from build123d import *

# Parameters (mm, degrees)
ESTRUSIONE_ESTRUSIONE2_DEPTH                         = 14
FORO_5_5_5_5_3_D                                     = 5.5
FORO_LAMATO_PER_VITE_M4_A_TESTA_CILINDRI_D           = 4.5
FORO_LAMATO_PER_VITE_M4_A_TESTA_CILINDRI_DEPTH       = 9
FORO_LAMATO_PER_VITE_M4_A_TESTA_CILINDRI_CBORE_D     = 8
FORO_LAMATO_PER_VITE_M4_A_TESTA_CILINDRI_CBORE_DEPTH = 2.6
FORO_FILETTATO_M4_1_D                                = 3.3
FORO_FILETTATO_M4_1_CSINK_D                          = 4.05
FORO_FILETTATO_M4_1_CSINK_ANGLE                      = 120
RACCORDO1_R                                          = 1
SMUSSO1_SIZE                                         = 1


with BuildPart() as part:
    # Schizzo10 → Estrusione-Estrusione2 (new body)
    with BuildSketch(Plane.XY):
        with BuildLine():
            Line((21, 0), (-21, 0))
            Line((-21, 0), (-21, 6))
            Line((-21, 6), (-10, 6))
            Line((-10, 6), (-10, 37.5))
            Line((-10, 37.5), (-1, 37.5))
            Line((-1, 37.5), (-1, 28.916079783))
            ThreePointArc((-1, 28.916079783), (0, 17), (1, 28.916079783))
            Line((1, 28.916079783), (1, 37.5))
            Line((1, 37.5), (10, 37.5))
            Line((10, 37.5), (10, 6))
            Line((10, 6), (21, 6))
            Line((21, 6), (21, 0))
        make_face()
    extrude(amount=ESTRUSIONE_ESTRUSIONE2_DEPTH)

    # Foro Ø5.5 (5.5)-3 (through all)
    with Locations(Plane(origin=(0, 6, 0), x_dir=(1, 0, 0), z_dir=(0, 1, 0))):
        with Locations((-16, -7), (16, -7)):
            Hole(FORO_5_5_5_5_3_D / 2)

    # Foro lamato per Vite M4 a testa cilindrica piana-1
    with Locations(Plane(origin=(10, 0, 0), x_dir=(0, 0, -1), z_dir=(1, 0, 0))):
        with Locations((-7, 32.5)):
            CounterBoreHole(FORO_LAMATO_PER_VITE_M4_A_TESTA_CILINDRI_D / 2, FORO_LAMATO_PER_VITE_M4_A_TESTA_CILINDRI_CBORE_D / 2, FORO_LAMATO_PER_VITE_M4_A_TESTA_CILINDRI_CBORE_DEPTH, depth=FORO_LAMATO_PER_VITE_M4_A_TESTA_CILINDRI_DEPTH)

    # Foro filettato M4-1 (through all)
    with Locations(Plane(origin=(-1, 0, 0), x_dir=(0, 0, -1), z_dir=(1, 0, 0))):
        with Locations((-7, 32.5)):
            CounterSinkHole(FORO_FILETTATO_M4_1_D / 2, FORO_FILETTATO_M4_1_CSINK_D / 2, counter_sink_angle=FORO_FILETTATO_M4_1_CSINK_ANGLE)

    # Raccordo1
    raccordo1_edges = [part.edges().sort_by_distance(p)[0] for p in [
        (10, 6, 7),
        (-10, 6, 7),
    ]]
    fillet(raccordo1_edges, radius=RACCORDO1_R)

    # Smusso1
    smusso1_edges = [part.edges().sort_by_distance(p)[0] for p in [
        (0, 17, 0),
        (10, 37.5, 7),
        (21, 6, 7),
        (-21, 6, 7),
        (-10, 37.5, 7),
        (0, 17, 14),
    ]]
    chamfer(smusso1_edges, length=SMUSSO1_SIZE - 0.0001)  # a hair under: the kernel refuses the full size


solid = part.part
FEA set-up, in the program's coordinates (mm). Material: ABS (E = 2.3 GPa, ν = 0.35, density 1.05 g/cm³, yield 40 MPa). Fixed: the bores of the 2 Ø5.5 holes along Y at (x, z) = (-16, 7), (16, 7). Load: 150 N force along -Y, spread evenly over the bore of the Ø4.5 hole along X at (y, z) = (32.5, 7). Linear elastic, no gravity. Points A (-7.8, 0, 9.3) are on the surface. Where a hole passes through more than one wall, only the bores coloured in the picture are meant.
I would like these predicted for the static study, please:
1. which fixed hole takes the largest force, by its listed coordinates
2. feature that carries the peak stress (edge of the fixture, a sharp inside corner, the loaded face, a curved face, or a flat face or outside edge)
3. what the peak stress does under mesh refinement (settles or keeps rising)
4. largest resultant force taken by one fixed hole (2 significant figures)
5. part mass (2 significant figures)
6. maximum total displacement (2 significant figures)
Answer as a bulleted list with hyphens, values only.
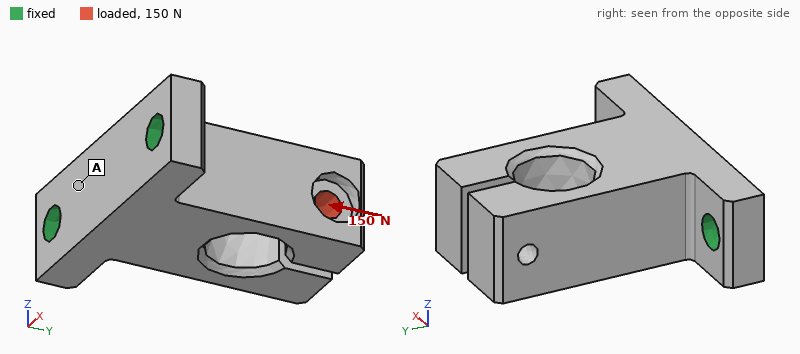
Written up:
- (16, 7)
- a sharp inside corner
- keeps rising
- 110 N
- 10 g
- 0.43 mm
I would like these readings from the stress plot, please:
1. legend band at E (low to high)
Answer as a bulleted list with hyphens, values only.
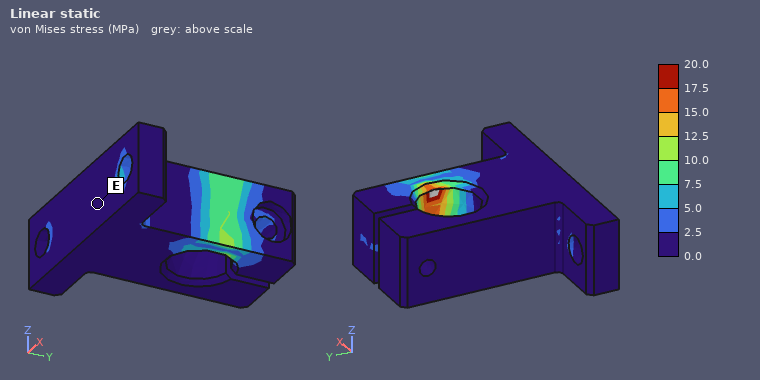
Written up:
- 0.0 to 2.5 MPa
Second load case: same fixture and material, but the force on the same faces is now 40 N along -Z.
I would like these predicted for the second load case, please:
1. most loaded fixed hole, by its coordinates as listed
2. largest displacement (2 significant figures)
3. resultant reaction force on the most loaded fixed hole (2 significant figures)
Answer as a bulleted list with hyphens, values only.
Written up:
- (16, 7)
- 0.31 mm
- 25 N
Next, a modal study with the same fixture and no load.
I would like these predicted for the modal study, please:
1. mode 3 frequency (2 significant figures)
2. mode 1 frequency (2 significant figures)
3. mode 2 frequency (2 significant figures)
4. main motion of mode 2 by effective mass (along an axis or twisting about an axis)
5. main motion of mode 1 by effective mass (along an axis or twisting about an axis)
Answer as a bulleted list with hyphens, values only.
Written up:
- 1800 Hz
- 1300 Hz
- 1600 Hz
- along X
- along Z
